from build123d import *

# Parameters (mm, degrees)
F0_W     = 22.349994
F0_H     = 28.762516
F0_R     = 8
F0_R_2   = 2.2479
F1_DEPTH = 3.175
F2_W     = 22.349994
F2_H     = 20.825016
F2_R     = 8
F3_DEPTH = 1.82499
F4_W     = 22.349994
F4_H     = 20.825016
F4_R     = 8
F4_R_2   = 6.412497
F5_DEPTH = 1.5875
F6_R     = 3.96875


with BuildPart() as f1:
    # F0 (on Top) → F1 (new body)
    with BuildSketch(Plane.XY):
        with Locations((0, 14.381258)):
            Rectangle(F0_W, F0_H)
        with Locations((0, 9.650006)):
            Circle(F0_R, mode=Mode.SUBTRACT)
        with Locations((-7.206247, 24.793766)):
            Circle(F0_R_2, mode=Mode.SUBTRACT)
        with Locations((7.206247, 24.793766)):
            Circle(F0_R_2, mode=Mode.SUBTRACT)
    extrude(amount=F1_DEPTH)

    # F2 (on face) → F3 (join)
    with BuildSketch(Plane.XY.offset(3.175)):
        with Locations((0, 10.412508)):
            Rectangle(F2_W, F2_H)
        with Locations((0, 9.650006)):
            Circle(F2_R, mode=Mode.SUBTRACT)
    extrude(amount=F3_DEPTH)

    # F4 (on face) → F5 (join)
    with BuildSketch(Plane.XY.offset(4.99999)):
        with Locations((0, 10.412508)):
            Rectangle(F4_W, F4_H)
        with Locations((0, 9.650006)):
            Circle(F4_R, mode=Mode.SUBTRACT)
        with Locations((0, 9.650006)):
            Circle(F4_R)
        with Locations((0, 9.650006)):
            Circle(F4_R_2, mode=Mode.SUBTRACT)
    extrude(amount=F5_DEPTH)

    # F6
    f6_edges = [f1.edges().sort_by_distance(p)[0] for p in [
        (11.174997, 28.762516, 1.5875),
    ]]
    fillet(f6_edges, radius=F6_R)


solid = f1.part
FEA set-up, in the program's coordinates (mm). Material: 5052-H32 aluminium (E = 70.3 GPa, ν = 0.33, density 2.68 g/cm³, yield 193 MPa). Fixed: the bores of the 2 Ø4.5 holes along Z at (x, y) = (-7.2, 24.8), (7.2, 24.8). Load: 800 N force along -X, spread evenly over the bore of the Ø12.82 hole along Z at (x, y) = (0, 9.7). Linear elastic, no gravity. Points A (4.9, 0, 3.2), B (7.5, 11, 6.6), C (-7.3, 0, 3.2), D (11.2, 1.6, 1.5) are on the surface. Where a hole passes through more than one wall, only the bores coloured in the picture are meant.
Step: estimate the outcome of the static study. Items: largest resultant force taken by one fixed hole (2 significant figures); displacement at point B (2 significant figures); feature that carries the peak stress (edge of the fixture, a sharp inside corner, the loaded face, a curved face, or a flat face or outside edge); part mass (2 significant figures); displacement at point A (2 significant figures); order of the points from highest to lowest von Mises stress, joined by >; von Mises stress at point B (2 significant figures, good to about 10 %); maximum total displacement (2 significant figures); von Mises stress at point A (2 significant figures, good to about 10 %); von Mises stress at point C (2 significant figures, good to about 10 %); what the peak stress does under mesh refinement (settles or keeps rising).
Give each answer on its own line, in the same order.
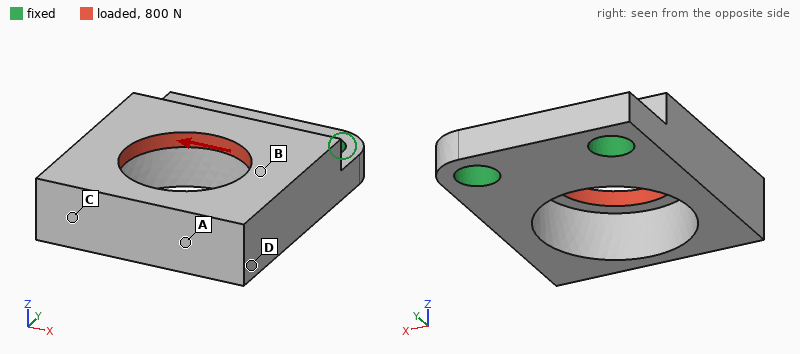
790 N
19 µm
edge of the fixture
6.2 g
36 µm
B > A > C > D
45 MPa
40 µm
30 MPa
18 MPa
keeps rising
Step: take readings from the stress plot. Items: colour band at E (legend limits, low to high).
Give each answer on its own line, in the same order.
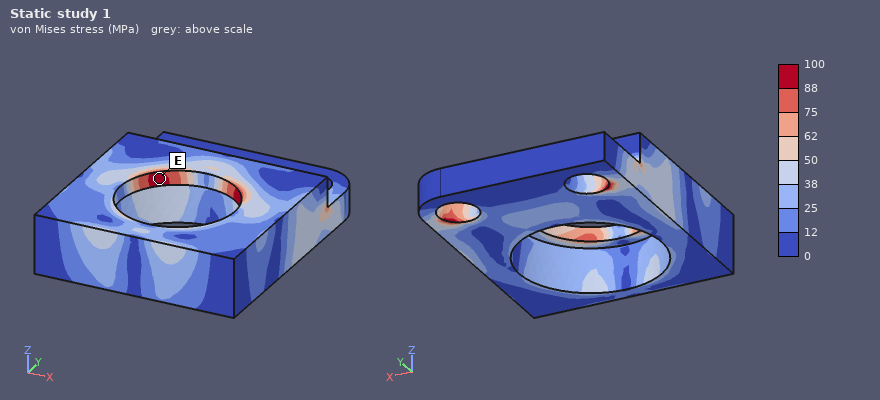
88 to 100 MPa
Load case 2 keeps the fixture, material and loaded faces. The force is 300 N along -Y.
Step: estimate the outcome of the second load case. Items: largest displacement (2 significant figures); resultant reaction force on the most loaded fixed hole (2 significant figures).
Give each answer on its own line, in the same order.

33 µm
150 N
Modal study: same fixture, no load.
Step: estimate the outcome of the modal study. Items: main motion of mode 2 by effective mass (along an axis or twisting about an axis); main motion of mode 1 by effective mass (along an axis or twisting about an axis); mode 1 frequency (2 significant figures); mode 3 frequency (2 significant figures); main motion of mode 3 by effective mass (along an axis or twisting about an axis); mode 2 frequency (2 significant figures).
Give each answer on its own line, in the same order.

along X
along Z
4900 Hz
14 kHz
along X
10 kHz
